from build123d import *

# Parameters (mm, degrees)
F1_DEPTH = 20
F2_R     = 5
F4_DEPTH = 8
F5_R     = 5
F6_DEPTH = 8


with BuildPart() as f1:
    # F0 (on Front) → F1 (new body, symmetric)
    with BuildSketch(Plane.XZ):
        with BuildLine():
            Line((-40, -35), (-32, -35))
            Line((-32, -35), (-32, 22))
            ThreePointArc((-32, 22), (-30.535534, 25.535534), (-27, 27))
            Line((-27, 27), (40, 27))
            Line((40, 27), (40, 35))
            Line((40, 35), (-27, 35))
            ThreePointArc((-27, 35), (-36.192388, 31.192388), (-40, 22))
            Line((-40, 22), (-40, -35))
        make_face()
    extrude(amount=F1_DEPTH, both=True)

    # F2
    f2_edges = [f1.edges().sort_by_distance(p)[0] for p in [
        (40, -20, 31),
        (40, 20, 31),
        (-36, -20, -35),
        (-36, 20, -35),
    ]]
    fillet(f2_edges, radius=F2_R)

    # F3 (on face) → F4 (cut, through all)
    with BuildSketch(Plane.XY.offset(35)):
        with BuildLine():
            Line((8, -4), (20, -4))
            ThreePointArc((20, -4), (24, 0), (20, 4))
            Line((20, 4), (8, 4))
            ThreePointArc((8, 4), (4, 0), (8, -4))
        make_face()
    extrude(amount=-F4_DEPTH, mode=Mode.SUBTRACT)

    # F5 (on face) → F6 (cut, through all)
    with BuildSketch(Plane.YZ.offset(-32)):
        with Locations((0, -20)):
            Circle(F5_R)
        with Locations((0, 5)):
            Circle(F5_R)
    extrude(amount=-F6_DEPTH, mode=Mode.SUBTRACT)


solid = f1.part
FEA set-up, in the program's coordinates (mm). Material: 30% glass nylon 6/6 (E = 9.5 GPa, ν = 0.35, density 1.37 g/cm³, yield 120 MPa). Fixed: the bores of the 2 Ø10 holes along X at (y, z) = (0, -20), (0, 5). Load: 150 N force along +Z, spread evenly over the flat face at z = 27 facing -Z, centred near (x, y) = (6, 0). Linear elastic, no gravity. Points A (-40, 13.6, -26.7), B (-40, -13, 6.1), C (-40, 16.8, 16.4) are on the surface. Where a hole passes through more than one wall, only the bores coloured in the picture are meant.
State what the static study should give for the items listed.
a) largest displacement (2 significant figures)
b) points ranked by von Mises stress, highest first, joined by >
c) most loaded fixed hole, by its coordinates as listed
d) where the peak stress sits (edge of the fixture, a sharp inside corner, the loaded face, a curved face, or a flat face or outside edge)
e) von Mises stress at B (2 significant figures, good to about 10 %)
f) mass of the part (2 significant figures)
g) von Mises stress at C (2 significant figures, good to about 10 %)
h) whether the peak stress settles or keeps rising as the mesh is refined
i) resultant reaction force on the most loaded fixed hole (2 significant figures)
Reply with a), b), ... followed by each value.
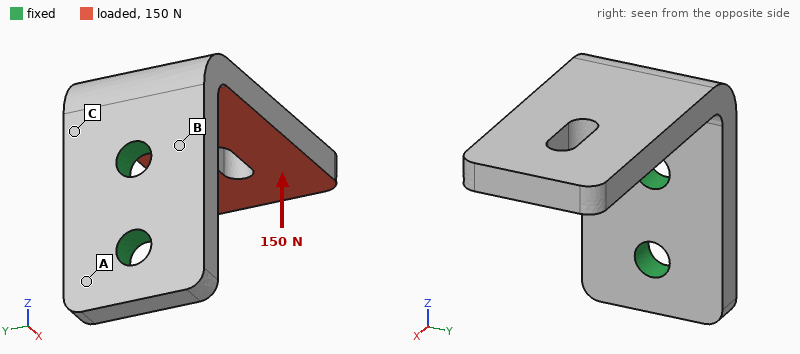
a) 1.1 mm
b) C > B > A
c) (0, 5)
d) edge of the fixture
e) 6.8 MPa
f) 57 g
g) 13 MPa
h) keeps rising
i) 150 N
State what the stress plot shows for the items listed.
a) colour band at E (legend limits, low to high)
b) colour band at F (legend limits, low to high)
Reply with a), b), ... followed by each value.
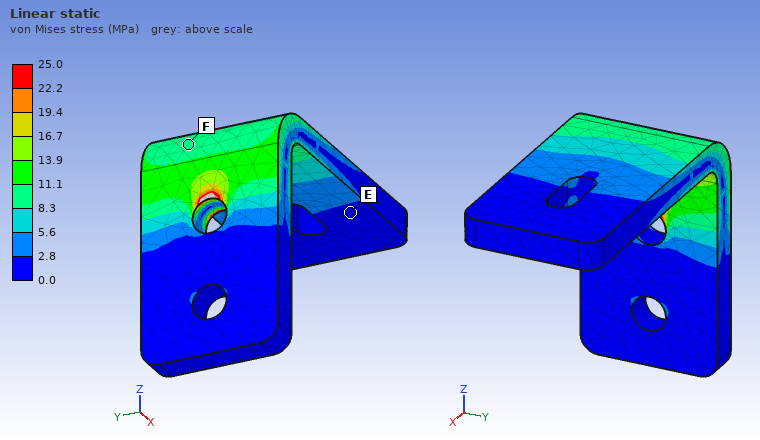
a) 0.0 to 2.8 MPa
b) 8.3 to 11.1 MPa
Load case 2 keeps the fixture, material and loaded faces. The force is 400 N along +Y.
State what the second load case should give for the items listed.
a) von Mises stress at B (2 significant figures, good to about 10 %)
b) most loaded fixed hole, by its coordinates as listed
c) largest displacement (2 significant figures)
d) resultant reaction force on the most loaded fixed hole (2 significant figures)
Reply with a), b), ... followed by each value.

a) 21 MPa
b) (0, 5)
c) 1.2 mm
d) 580 N
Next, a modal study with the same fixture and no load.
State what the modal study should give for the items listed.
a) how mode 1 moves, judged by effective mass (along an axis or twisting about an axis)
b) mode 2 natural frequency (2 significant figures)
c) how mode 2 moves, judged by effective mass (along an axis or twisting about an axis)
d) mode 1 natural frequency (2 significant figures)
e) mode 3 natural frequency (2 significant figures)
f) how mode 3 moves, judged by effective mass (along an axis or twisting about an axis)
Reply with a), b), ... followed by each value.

a) along Z
b) 670 Hz
c) along Y
d) 420 Hz
e) 1900 Hz
f) along X
